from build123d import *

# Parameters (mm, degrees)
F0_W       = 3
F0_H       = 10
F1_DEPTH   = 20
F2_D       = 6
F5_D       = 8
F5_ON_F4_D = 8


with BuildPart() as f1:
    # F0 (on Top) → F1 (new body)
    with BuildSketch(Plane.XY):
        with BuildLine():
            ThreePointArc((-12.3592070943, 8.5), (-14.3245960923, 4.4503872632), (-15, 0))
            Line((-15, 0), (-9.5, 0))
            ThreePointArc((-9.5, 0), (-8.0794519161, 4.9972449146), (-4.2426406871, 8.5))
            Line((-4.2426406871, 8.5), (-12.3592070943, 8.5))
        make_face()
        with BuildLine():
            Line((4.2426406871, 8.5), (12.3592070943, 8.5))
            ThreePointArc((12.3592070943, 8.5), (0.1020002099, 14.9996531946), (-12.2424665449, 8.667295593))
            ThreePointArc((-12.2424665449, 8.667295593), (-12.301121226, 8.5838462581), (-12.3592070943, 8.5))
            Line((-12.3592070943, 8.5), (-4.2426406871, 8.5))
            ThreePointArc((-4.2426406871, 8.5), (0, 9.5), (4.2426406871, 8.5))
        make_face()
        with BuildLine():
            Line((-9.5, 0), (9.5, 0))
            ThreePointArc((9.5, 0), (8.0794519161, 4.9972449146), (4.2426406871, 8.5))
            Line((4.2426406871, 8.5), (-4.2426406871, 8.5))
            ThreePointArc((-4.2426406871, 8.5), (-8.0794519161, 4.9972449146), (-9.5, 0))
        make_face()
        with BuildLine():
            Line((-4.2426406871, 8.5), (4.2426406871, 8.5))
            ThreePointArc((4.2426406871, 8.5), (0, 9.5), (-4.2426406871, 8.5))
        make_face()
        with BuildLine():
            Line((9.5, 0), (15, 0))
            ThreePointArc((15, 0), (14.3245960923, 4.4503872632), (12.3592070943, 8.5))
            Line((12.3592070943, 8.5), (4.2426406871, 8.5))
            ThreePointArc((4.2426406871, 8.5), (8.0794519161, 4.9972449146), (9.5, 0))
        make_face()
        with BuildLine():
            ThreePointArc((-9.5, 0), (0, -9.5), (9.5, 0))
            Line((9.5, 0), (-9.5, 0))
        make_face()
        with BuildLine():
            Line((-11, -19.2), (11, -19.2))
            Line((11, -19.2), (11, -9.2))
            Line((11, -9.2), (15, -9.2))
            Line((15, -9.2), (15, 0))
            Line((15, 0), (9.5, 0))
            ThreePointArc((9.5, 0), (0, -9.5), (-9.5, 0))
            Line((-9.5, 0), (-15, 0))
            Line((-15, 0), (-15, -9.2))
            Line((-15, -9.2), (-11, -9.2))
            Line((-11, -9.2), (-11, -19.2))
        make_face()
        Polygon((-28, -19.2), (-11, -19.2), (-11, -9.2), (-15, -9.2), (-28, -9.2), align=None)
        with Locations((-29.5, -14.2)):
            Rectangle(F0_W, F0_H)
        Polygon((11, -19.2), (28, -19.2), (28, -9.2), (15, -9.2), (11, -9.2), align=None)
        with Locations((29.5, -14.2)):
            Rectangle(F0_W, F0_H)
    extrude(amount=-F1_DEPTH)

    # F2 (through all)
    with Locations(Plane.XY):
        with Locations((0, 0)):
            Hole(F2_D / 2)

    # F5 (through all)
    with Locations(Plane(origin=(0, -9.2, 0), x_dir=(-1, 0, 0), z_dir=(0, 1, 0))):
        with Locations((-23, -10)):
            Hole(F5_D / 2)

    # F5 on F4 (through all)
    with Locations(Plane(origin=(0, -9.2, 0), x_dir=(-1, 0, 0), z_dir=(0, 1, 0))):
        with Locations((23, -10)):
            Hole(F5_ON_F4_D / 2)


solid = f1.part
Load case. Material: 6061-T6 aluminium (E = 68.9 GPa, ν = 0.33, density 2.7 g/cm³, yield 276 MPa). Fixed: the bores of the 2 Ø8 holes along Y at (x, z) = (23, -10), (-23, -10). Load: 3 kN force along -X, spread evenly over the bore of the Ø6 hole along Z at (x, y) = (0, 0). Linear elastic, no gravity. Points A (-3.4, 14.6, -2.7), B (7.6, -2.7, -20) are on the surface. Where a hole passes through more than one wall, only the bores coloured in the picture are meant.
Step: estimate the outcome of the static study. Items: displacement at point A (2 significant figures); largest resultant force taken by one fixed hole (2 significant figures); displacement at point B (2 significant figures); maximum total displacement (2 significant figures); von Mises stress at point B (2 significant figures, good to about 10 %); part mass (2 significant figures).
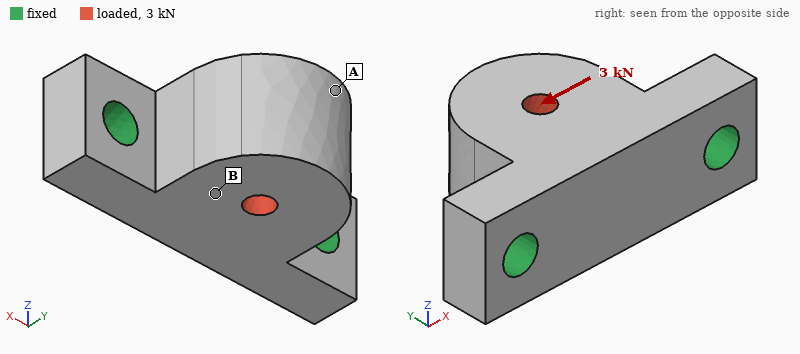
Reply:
8.5 µm
1.9 kN
4.5 µm
8.6 µm
11 MPa
63 g
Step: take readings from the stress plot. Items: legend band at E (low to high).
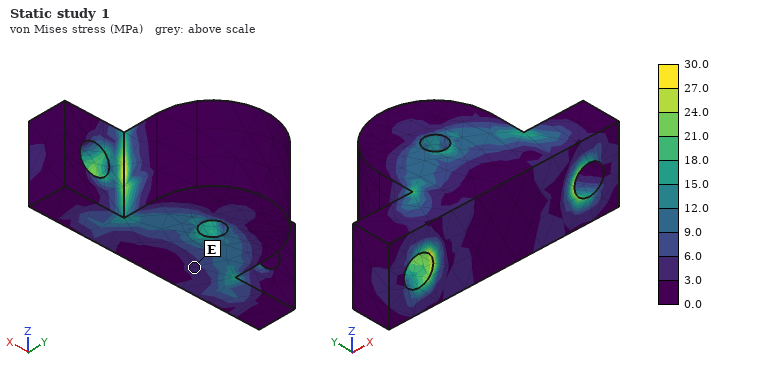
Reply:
3.0 to 6.0 MPa
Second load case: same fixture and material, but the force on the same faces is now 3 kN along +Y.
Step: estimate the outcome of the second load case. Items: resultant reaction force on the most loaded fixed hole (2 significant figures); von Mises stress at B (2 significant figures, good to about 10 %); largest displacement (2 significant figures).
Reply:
1.6 kN
6.2 MPa
6.3 µm
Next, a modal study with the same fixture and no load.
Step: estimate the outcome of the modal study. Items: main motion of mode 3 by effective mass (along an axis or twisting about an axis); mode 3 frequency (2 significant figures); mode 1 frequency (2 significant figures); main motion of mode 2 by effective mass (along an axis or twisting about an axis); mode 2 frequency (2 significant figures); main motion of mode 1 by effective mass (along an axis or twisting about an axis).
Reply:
along Y
18 kHz
7500 Hz
along X
17 kHz
along Z
